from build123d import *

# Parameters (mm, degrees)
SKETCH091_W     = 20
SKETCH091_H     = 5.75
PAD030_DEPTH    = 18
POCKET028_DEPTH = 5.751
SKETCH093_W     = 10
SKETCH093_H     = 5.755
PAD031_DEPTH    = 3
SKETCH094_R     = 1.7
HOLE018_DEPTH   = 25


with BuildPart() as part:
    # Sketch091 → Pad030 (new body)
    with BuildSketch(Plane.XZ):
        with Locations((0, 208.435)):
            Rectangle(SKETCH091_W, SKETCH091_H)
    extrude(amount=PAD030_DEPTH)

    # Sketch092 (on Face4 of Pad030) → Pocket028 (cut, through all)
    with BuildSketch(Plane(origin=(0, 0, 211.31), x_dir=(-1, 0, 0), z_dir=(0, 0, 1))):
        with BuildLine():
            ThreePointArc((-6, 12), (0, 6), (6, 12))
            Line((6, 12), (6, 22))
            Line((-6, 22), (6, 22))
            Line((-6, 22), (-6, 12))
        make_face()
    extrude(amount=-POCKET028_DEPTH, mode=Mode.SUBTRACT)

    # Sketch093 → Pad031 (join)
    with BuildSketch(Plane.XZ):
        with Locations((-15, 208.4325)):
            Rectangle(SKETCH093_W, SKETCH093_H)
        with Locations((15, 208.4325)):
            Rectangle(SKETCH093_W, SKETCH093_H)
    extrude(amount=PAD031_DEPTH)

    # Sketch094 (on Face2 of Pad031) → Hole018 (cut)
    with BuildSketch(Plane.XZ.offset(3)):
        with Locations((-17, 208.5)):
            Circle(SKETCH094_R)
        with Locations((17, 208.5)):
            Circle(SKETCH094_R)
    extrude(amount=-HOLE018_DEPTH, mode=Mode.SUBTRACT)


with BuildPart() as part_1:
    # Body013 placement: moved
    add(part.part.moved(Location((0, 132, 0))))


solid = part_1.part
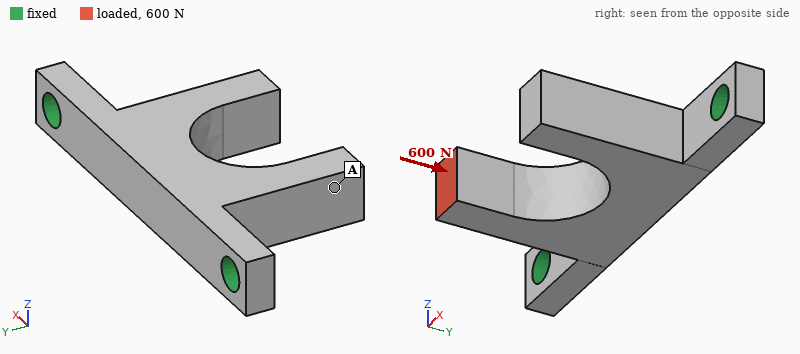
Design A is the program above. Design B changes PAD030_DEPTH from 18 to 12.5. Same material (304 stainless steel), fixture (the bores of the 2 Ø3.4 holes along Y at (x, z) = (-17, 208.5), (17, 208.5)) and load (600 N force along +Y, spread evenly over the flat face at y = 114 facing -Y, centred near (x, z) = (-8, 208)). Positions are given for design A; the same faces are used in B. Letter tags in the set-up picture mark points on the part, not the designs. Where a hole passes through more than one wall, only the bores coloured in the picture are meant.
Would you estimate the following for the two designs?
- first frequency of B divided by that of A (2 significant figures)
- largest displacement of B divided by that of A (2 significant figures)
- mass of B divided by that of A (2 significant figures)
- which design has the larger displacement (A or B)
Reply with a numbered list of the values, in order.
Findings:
1. 1.6
2. 0.91
3. 0.84
4. A
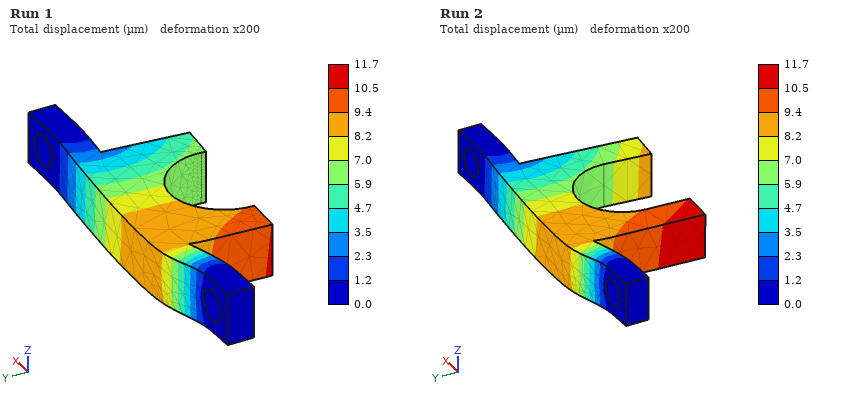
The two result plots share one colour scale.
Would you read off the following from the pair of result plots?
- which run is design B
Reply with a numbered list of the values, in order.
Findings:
1. Run 1
